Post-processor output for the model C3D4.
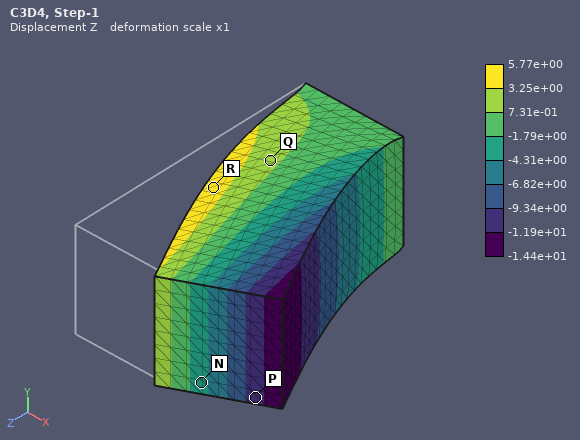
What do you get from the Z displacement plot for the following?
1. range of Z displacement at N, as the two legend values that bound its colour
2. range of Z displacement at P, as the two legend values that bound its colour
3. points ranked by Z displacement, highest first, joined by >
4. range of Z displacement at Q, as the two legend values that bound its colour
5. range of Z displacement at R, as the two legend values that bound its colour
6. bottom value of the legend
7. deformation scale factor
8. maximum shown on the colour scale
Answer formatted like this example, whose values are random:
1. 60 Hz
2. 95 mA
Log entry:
1. -4.31e+00 to -1.79e+00
2. -1.19e+01 to -9.34e+00
3. R > Q > N > P
4. 7.31e-01 to 3.25e+00
5. 3.25e+00 to 5.77e+00
6. -1.44e+01
7. 1
8. 5.77e+00
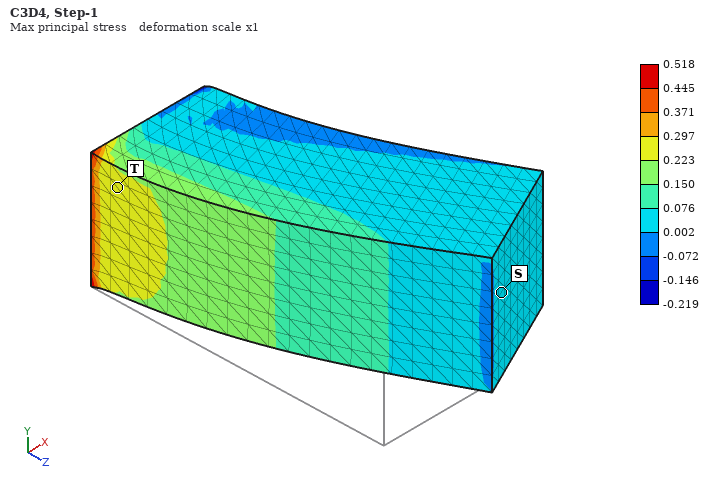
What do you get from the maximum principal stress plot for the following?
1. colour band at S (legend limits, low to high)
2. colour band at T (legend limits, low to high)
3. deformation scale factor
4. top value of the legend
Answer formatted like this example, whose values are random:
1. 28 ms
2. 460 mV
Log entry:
1. 0.002 to 0.076
2. 0.223 to 0.297
3. 1
4. 0.518
